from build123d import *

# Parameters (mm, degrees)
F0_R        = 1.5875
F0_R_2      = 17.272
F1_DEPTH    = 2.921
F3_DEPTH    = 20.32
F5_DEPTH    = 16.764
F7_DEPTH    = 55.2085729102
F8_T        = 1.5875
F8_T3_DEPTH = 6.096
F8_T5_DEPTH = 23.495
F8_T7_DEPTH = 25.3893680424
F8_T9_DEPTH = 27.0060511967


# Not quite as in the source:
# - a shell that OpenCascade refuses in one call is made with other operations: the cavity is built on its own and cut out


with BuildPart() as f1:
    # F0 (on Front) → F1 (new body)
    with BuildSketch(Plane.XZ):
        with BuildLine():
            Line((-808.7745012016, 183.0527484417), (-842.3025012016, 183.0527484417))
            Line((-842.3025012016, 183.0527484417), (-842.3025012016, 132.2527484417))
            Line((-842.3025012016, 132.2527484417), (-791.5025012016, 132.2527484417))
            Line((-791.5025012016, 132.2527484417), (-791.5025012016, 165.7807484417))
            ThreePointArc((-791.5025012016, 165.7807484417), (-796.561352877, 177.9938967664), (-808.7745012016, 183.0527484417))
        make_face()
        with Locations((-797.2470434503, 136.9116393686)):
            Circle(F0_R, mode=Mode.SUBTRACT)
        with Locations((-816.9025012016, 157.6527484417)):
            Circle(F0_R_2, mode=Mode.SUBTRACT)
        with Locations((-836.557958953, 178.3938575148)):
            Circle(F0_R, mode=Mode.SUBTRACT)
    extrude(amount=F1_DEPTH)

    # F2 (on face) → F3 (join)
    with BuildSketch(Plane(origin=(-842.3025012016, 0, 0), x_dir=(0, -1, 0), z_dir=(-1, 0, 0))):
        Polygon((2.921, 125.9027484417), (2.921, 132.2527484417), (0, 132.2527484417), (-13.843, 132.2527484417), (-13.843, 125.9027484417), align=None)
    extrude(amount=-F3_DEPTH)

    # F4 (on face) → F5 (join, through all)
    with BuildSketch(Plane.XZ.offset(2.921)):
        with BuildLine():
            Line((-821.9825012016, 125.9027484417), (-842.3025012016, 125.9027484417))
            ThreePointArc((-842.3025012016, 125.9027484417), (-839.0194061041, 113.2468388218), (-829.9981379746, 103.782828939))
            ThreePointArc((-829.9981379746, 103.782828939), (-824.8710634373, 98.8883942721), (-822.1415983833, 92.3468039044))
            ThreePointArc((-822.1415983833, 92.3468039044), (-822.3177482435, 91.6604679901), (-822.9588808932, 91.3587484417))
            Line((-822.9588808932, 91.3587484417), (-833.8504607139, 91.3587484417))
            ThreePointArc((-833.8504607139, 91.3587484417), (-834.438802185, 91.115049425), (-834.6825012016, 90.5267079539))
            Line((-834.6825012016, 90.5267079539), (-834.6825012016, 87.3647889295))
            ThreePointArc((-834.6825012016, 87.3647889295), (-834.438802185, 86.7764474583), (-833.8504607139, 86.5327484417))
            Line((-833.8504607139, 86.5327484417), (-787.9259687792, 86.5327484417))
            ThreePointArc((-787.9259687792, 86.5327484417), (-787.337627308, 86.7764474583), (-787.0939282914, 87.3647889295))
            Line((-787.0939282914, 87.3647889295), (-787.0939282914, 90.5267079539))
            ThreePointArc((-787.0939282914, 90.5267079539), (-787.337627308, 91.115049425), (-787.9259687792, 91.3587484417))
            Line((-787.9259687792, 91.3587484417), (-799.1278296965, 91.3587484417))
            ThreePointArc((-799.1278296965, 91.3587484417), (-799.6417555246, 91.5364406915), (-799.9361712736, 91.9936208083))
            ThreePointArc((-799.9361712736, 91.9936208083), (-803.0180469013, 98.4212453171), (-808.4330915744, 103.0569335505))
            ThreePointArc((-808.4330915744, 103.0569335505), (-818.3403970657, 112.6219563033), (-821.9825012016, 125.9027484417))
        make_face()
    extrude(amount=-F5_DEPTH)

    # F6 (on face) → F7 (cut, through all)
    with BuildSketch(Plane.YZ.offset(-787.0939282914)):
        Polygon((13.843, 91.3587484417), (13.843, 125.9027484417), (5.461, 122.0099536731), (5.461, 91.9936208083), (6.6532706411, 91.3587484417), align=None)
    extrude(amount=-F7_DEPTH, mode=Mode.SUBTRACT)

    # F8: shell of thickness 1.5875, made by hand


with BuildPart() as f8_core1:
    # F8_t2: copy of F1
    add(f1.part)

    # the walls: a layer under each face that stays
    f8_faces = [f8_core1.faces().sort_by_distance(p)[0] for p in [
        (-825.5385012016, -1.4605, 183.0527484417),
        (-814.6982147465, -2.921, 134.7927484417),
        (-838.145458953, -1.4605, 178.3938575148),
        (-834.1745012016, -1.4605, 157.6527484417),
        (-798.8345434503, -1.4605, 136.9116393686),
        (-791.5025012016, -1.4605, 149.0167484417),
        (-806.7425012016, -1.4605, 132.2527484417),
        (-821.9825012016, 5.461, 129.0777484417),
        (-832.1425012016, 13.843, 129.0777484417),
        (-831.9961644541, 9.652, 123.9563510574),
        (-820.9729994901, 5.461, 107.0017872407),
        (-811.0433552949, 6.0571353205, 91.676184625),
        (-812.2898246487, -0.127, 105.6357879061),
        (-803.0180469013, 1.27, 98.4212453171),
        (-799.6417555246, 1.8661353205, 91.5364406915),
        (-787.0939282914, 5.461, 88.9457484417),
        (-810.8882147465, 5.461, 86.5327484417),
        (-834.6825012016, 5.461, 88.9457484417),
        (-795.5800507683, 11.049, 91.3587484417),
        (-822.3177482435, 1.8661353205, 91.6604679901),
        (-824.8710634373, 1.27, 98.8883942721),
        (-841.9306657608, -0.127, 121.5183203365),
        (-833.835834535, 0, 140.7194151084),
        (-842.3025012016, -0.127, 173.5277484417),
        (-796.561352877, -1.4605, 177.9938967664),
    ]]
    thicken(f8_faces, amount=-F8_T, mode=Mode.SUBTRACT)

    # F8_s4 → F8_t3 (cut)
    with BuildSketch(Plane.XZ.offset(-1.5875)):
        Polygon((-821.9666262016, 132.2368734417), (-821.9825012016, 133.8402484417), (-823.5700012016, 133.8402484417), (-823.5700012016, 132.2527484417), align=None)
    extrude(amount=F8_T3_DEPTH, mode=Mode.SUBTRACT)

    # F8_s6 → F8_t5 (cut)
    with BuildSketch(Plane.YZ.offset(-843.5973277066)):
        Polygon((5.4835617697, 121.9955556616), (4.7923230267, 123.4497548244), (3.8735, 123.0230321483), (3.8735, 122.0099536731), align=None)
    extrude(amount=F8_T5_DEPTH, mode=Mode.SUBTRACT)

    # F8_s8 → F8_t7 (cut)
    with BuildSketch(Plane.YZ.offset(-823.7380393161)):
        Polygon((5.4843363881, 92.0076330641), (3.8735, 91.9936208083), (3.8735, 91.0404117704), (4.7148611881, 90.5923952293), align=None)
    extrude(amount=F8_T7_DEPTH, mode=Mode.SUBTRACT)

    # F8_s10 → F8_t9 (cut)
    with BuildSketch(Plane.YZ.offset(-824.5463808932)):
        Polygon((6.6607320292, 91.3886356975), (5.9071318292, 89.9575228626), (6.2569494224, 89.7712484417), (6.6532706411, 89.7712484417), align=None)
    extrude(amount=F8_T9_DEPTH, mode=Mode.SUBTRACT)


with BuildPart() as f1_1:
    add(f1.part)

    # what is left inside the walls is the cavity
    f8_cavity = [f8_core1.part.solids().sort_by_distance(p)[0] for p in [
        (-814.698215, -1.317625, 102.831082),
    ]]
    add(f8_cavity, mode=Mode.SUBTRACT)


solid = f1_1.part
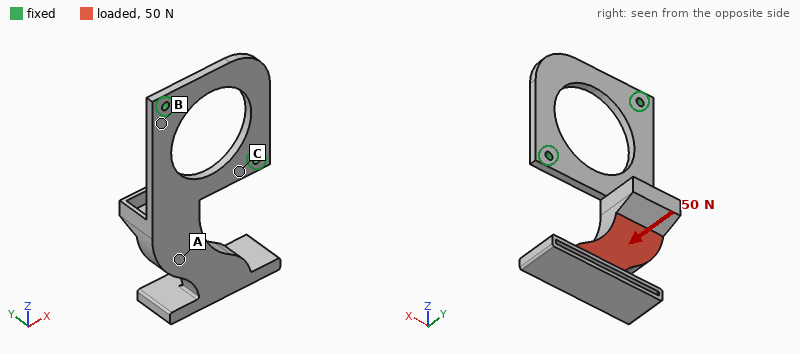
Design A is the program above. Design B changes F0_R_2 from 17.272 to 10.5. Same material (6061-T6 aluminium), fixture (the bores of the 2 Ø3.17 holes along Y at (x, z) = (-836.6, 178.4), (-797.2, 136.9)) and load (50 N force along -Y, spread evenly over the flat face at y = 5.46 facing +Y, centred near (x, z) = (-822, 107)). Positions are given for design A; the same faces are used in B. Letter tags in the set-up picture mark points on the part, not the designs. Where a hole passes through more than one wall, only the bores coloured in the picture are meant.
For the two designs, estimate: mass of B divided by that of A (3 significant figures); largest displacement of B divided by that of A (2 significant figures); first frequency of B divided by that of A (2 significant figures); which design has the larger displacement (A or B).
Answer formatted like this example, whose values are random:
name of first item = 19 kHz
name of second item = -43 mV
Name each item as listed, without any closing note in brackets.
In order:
mass of B divided by that of A = 1.16
largest displacement of B divided by that of A = 0.78
first frequency of B divided by that of A = 1.1
which design has the larger displacement = A
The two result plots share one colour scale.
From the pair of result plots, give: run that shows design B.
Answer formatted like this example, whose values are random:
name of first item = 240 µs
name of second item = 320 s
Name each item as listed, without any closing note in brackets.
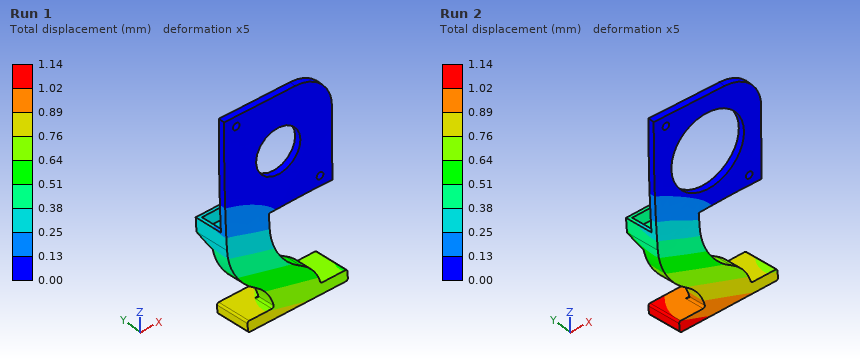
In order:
run that shows design B = Run 1
